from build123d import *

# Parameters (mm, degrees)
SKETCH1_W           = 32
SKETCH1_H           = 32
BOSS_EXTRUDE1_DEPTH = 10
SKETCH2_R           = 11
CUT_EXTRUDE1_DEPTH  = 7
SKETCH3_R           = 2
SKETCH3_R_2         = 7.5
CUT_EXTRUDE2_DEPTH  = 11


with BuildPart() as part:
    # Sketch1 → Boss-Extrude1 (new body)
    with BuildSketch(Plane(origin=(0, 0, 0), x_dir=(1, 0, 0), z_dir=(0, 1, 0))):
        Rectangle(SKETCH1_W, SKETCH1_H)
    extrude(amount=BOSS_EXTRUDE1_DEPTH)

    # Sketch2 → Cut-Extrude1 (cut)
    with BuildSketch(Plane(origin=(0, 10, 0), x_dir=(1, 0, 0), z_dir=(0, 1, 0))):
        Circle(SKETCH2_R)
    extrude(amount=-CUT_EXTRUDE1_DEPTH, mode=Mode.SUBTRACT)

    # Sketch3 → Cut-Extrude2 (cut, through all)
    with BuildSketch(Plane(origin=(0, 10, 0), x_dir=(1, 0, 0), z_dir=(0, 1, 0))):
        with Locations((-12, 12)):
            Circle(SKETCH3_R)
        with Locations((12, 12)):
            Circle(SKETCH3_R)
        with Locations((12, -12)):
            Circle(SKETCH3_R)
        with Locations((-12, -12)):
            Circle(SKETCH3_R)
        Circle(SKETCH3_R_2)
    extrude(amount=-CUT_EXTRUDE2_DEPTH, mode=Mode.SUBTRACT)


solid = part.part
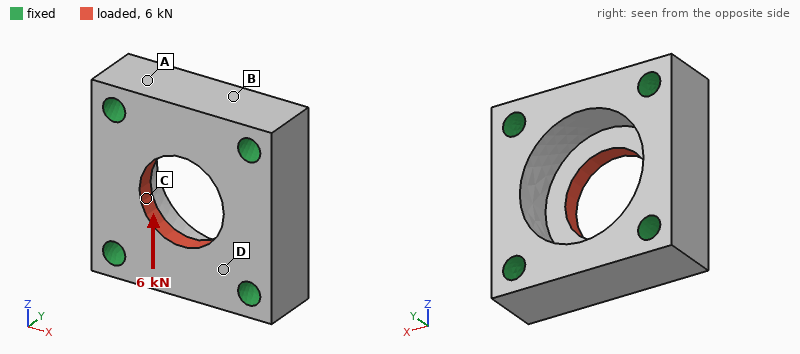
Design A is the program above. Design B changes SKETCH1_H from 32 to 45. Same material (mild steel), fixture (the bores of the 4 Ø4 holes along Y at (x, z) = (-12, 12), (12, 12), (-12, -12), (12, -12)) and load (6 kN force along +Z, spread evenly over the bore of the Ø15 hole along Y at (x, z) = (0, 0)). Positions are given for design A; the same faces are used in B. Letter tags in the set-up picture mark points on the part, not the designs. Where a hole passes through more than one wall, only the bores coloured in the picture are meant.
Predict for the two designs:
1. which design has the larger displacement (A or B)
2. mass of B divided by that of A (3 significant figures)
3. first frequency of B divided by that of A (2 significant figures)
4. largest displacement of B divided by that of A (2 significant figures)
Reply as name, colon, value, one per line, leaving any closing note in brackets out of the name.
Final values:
which design has the larger displacement: A
mass of B divided by that of A: 1.64
first frequency of B divided by that of A: 0.84
largest displacement of B divided by that of A: 0.74
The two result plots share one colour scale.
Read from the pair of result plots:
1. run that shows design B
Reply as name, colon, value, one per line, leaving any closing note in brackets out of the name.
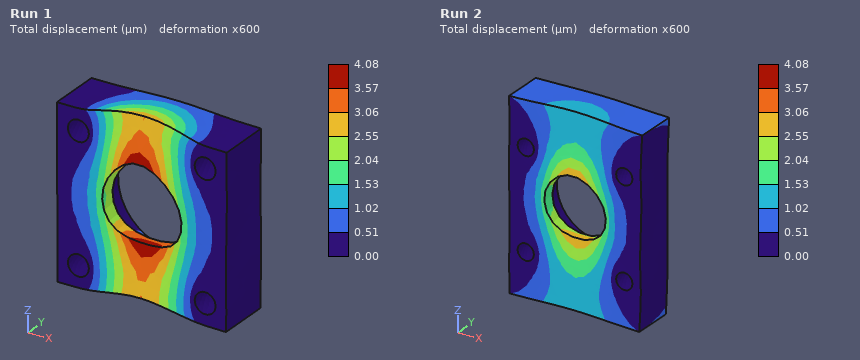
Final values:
run that shows design B: Run 2
